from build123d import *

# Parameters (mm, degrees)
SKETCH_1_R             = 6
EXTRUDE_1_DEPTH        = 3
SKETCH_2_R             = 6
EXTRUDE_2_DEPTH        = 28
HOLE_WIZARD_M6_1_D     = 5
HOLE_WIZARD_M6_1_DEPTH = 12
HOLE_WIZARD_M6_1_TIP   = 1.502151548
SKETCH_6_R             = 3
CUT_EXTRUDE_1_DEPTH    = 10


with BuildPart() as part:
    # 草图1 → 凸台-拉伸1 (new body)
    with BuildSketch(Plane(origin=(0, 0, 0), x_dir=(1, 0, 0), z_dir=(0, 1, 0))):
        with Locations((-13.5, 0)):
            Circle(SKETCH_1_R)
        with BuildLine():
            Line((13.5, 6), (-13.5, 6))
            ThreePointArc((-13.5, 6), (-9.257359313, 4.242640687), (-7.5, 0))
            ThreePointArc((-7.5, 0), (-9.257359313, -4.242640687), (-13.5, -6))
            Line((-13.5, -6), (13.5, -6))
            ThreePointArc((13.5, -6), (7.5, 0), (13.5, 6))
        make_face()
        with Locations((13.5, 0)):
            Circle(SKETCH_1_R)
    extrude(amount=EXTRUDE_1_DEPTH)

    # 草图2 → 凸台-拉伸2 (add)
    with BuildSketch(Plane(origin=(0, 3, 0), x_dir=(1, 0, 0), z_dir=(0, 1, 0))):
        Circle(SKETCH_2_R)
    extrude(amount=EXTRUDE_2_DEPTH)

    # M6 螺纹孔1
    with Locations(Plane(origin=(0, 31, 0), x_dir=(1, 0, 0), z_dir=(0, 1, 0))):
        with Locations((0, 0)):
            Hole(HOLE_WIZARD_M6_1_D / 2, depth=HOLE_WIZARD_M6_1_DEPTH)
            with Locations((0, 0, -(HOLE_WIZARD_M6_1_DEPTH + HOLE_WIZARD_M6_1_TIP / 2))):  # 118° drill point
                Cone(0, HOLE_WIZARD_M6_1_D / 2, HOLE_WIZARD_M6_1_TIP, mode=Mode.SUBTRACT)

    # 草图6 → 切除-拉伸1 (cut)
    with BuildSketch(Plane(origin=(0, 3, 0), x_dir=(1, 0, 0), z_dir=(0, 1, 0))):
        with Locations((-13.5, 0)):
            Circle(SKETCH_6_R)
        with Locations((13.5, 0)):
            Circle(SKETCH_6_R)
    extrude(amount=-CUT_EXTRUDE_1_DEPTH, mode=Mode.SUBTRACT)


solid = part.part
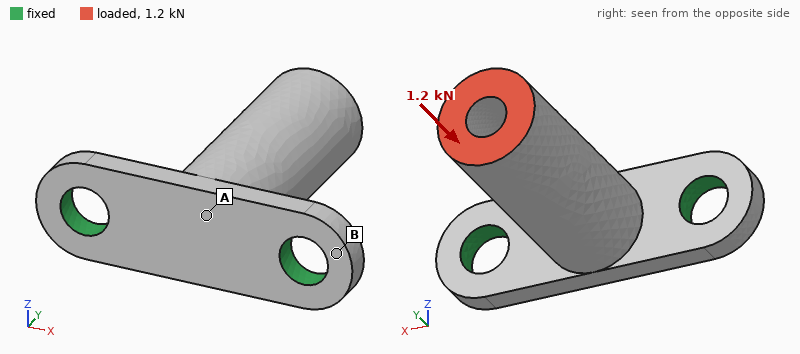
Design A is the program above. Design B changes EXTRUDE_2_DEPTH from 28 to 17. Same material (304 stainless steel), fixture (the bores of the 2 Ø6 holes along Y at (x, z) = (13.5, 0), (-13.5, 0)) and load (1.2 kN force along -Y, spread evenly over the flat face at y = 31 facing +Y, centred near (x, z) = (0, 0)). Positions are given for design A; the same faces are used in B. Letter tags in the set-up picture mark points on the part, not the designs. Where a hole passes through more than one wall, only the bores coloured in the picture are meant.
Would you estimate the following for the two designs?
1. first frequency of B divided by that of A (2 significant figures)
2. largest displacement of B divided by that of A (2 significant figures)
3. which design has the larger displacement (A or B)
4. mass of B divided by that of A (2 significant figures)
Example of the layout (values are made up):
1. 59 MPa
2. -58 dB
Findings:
1. 1.9
2. 0.91
3. A
4. 0.75
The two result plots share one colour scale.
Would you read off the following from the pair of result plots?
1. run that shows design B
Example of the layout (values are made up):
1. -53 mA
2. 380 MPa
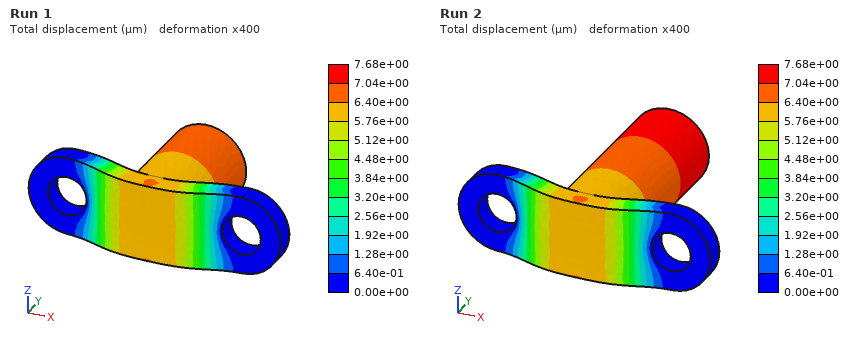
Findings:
1. Run 1
